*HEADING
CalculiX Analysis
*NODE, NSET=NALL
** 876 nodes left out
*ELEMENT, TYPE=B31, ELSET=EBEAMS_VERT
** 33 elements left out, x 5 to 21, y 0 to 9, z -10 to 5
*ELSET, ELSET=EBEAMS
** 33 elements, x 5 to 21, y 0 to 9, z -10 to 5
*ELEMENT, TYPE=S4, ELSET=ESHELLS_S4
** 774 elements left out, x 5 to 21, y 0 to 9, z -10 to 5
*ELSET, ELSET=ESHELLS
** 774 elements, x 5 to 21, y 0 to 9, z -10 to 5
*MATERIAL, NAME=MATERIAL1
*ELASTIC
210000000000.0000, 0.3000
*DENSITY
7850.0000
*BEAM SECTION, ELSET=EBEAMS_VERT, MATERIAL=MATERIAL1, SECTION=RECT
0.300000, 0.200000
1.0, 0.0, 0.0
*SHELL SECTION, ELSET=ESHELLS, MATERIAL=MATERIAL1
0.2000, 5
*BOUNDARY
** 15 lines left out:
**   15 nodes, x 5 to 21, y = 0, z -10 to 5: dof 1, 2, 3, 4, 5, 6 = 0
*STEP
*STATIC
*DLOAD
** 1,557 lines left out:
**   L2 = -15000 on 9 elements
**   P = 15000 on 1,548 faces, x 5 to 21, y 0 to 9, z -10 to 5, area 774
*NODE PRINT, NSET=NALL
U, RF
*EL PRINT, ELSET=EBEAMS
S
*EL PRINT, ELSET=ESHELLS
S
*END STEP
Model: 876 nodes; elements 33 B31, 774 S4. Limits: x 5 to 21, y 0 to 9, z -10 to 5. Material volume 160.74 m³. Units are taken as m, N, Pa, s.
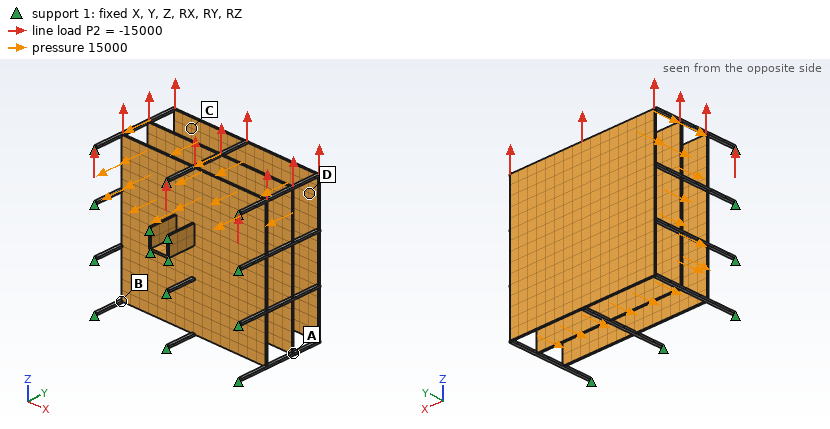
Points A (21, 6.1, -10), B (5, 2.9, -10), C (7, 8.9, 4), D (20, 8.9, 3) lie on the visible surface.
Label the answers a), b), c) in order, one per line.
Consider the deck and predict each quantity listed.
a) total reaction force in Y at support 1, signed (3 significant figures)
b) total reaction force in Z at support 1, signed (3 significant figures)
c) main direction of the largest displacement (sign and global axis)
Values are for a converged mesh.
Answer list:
a) 2.16e+07 N
b) -9.45e+05 N
c) -Y
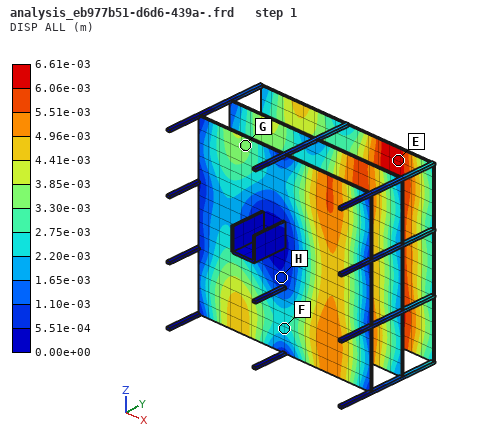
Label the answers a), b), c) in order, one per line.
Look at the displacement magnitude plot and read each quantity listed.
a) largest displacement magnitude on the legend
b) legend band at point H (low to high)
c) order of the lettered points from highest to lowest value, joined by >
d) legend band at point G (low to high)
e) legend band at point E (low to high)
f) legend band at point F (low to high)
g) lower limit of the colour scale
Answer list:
a) 6.61e-03 m
b) 5.51e-04 to 1.10e-03 m
c) E > G > F > H
d) 3.30e-03 to 3.85e-03 m
e) 6.06e-03 to 6.61e-03 m
f) 2.20e-03 to 2.75e-03 m
g) 0.00e+00 m
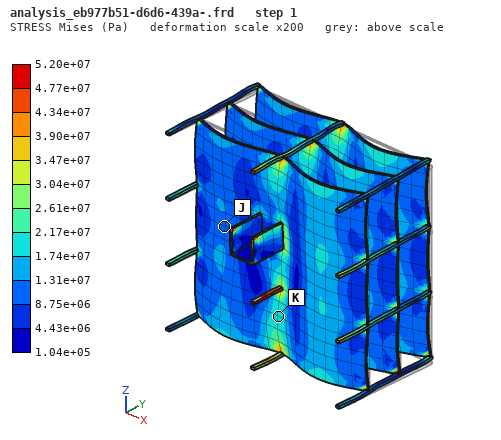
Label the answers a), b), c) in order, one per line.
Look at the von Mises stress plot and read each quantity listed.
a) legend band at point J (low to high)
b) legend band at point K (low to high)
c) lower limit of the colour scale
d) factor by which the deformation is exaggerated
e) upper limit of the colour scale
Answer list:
a) 8.75e+06 to 1.31e+07 Pa
b) 1.74e+07 to 2.17e+07 Pa
c) 1.04e+05 Pa
d) 200
e) 5.20e+07 Pa
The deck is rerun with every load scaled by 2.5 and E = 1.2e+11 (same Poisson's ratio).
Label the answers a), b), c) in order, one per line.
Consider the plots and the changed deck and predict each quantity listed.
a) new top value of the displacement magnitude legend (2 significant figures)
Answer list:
a) 0.029 m
